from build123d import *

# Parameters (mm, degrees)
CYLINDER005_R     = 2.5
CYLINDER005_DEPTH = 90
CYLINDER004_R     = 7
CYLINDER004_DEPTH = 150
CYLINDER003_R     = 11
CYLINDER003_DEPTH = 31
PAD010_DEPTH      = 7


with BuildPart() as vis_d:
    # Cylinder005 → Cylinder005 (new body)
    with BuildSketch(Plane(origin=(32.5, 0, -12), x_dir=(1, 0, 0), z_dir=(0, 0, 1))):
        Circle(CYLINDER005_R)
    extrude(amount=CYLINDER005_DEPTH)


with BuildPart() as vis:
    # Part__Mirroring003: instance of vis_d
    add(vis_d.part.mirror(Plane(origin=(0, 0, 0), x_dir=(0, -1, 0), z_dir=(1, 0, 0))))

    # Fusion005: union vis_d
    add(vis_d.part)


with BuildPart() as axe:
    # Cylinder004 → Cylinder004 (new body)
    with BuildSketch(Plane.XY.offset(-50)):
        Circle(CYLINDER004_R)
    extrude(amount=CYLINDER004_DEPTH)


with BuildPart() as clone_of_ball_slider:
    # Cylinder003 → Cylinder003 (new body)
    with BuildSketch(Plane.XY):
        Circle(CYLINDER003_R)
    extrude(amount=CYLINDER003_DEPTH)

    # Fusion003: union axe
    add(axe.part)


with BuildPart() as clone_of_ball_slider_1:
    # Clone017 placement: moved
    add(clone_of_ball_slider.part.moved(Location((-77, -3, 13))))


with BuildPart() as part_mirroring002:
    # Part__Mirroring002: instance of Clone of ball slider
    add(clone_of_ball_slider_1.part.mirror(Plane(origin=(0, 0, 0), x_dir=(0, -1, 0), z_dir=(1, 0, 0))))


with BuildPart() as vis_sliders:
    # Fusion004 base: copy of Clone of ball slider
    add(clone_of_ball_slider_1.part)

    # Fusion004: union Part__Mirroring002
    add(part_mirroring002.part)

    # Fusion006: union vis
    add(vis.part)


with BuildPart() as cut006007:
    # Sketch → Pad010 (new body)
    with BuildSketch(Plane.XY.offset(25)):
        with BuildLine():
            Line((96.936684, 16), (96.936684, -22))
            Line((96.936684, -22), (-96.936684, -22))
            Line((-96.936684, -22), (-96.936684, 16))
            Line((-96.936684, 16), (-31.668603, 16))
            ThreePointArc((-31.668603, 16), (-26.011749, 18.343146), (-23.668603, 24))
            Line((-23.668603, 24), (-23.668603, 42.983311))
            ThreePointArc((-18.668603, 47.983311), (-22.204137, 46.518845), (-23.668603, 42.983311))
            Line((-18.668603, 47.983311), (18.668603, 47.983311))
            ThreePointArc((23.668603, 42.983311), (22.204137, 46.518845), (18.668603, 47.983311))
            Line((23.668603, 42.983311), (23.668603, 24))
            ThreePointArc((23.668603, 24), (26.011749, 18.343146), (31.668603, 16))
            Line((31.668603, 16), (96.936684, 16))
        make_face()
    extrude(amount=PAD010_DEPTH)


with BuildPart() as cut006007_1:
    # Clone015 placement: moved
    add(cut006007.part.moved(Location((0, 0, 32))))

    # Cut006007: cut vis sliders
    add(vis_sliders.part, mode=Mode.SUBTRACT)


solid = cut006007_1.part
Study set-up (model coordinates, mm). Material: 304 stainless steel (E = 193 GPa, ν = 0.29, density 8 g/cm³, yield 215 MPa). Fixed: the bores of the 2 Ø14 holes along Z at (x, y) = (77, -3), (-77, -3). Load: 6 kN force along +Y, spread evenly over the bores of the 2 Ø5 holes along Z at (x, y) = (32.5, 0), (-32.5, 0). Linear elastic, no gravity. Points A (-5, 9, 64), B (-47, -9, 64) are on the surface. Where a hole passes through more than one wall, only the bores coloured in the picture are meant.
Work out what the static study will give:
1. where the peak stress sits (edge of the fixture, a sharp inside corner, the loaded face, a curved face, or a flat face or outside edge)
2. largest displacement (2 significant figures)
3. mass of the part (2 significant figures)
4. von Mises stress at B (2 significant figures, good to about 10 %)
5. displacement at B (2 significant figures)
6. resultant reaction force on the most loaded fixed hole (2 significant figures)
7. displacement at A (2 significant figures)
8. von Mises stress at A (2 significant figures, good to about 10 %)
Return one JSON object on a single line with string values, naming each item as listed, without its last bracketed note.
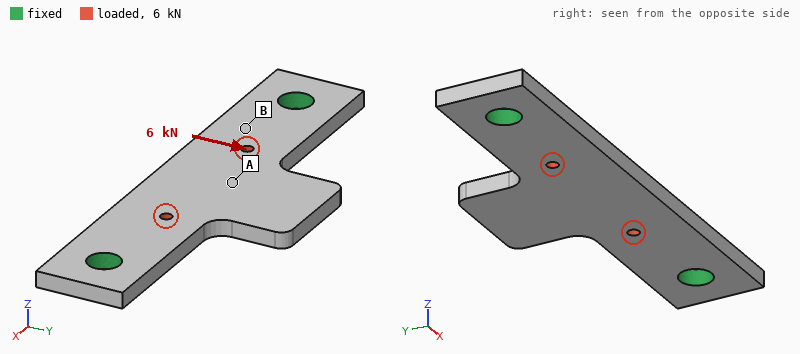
{"where the peak stress sits": "edge of the fixture", "largest displacement": "21 µm", "mass of the part": "480 g", "von Mises stress at B": "25 MPa", "displacement at B": "12 µm", "resultant reaction force on the most loaded fixed hole": "3.0 kN", "displacement at A": "20 µm", "von Mises stress at A": "12 MPa"}
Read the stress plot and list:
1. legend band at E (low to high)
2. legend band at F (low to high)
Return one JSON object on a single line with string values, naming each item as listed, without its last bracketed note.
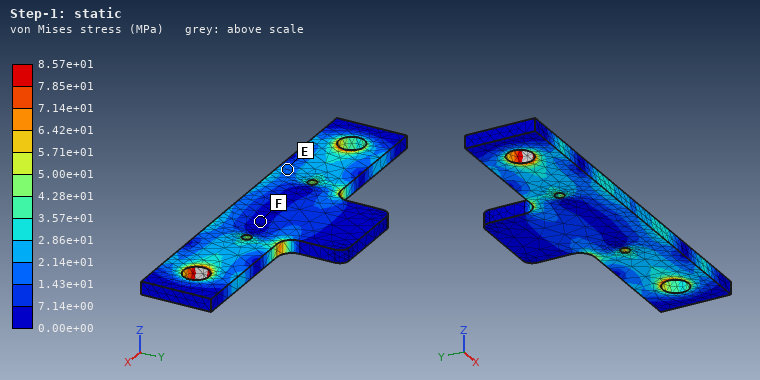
{"legend band at E": "1.43e+01 to 2.14e+01 MPa", "legend band at F": "0.00e+00 to 7.14e+00 MPa"}
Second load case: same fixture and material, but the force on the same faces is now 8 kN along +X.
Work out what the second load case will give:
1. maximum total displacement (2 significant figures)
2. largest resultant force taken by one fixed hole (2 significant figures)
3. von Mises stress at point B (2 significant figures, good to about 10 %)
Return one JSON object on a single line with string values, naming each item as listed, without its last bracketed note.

{"maximum total displacement": "4.9 µm", "largest resultant force taken by one fixed hole": "4.0 kN", "von Mises stress at point B": "17 MPa"}
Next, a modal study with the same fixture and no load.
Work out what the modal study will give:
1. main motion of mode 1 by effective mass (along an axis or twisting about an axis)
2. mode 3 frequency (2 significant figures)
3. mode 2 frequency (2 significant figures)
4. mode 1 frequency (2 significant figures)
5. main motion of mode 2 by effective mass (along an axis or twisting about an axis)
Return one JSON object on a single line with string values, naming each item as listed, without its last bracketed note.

{"main motion of mode 1 by effective mass": "along Z", "mode 3 frequency": "3900 Hz", "mode 2 frequency": "2100 Hz", "mode 1 frequency": "1100 Hz", "main motion of mode 2 by effective mass": "along Z"}
